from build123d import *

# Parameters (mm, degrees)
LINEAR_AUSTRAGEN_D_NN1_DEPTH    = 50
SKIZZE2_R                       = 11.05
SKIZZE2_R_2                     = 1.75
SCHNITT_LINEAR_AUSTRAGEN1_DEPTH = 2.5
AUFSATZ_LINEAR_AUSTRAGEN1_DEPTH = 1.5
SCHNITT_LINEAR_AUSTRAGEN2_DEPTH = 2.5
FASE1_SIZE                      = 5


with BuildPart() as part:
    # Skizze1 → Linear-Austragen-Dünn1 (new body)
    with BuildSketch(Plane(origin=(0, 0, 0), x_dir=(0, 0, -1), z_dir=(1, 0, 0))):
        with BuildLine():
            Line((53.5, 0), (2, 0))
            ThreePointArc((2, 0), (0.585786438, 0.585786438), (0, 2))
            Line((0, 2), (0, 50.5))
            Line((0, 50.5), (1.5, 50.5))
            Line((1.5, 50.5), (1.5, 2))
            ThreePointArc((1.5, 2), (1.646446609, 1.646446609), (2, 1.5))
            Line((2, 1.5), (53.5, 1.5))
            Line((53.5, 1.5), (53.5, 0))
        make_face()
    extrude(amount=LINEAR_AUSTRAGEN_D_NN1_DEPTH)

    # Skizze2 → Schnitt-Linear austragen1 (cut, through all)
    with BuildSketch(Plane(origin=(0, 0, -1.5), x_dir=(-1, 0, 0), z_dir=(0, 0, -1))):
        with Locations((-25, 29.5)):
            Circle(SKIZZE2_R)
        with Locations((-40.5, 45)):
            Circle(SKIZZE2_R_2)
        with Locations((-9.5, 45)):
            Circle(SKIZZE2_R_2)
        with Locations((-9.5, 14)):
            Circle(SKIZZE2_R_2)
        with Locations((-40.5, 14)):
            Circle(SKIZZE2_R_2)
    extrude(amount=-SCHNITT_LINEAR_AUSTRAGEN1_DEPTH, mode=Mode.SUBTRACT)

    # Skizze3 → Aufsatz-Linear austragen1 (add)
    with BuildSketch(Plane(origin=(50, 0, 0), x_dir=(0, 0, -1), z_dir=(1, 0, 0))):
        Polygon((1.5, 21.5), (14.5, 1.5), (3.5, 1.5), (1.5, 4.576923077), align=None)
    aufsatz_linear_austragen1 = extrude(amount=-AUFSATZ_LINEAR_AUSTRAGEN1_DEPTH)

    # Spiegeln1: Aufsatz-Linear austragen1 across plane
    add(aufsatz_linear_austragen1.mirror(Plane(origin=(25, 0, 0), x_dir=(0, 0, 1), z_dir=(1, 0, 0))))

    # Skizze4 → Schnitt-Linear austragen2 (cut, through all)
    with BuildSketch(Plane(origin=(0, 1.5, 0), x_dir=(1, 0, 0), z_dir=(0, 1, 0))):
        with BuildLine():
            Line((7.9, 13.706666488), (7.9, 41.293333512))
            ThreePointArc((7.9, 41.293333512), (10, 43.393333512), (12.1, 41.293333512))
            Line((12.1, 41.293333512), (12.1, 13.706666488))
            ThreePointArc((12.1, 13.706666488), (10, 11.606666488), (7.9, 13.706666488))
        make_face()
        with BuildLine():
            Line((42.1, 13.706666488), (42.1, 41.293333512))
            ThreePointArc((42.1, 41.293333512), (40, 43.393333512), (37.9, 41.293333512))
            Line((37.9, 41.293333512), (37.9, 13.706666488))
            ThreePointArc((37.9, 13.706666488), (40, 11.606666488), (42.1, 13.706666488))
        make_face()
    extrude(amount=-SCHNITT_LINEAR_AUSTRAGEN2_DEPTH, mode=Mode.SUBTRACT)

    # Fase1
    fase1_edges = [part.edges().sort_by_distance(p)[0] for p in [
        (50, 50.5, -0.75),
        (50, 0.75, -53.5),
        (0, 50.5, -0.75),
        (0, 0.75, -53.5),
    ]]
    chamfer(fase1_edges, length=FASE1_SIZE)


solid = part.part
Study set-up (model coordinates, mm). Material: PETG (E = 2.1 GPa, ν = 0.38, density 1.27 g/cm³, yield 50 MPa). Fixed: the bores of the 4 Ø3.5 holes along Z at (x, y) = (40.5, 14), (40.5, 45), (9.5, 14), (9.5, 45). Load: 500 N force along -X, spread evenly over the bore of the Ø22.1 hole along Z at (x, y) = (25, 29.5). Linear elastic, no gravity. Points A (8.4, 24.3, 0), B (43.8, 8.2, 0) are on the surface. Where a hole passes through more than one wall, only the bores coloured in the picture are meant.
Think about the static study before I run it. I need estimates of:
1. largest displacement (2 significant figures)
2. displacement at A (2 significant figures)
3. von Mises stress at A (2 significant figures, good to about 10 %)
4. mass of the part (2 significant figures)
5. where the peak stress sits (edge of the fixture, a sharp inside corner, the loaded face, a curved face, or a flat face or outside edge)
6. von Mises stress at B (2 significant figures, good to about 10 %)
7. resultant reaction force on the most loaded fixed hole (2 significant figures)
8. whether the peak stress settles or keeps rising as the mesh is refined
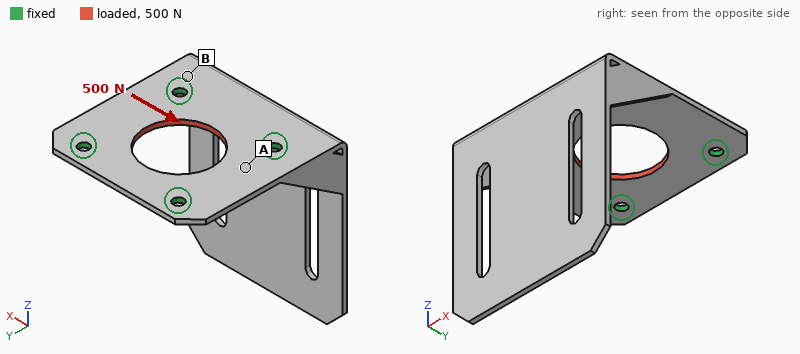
77 µm
56 µm
4.6 MPa
8.8 g
edge of the fixture
1.7 MPa
130 N
keeps rising
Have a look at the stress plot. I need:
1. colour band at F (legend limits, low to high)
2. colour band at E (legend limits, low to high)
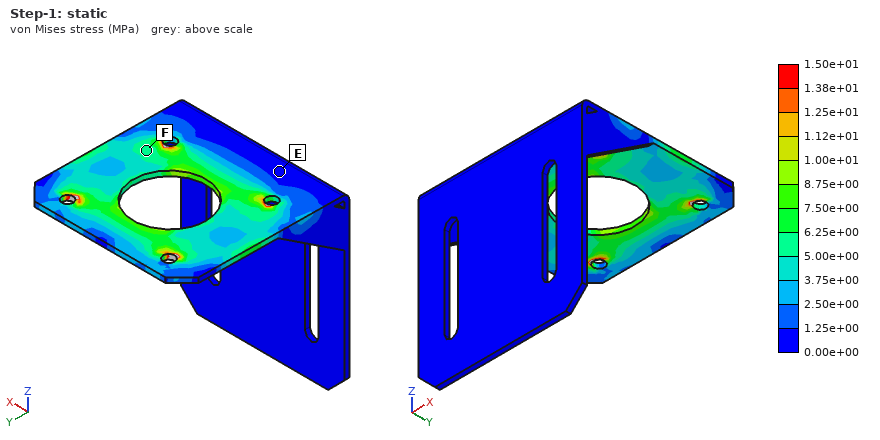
5.00e+00 to 6.25e+00 MPa
0.00e+00 to 1.25e+00 MPa
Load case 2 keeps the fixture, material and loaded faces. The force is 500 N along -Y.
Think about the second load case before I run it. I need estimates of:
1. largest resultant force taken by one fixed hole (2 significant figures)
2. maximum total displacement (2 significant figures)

130 N
0.10 mm
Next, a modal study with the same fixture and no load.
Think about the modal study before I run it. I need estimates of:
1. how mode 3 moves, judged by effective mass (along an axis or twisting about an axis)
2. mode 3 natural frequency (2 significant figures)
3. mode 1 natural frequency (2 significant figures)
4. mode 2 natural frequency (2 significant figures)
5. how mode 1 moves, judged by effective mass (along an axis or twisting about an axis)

along X
430 Hz
120 Hz
280 Hz
along Y
